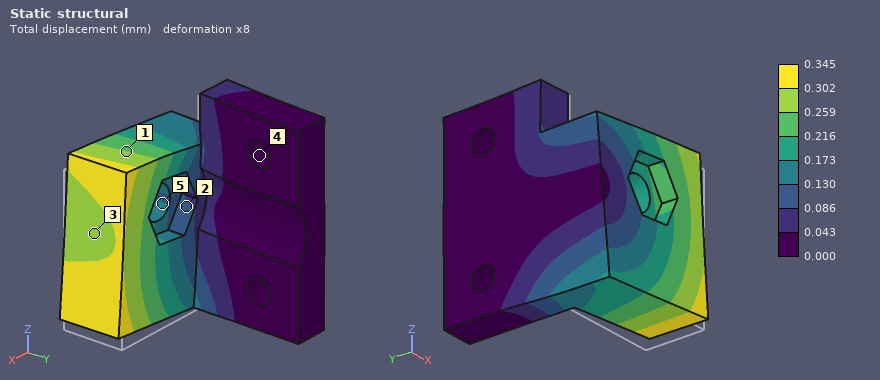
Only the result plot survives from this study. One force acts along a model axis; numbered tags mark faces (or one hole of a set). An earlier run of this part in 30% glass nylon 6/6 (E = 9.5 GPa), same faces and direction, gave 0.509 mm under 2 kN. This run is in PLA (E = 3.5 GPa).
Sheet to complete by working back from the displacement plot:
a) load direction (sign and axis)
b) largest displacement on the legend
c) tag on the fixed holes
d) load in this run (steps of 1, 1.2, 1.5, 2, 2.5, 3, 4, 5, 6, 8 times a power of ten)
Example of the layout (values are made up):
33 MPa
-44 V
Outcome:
+Z
0.345 mm
4
500 N
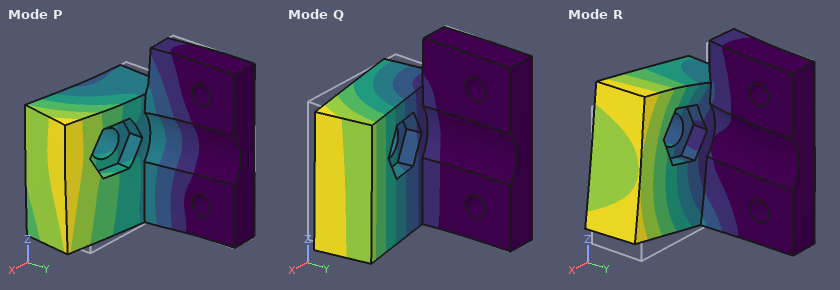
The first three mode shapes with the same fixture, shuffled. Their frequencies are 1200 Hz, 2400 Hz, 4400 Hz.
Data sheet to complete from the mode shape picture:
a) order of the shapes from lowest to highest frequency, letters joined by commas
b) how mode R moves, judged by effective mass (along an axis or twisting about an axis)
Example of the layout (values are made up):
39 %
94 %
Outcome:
Q, R, P
along Z
